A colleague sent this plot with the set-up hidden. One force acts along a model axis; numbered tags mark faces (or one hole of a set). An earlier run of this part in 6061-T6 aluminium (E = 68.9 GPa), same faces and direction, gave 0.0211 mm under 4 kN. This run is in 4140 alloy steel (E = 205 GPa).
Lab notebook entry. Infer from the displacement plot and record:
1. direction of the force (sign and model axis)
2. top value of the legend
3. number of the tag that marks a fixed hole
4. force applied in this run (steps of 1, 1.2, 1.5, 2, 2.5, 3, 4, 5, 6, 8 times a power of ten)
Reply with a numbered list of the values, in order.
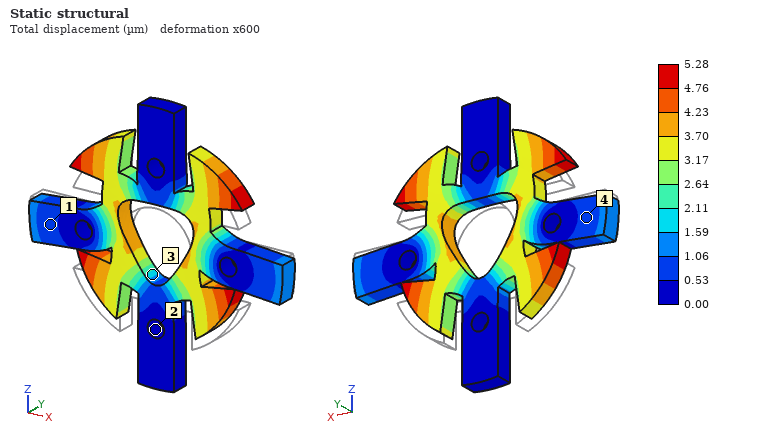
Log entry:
1. +Z
2. 5.28 µm
3. 2
4. 3 kN
